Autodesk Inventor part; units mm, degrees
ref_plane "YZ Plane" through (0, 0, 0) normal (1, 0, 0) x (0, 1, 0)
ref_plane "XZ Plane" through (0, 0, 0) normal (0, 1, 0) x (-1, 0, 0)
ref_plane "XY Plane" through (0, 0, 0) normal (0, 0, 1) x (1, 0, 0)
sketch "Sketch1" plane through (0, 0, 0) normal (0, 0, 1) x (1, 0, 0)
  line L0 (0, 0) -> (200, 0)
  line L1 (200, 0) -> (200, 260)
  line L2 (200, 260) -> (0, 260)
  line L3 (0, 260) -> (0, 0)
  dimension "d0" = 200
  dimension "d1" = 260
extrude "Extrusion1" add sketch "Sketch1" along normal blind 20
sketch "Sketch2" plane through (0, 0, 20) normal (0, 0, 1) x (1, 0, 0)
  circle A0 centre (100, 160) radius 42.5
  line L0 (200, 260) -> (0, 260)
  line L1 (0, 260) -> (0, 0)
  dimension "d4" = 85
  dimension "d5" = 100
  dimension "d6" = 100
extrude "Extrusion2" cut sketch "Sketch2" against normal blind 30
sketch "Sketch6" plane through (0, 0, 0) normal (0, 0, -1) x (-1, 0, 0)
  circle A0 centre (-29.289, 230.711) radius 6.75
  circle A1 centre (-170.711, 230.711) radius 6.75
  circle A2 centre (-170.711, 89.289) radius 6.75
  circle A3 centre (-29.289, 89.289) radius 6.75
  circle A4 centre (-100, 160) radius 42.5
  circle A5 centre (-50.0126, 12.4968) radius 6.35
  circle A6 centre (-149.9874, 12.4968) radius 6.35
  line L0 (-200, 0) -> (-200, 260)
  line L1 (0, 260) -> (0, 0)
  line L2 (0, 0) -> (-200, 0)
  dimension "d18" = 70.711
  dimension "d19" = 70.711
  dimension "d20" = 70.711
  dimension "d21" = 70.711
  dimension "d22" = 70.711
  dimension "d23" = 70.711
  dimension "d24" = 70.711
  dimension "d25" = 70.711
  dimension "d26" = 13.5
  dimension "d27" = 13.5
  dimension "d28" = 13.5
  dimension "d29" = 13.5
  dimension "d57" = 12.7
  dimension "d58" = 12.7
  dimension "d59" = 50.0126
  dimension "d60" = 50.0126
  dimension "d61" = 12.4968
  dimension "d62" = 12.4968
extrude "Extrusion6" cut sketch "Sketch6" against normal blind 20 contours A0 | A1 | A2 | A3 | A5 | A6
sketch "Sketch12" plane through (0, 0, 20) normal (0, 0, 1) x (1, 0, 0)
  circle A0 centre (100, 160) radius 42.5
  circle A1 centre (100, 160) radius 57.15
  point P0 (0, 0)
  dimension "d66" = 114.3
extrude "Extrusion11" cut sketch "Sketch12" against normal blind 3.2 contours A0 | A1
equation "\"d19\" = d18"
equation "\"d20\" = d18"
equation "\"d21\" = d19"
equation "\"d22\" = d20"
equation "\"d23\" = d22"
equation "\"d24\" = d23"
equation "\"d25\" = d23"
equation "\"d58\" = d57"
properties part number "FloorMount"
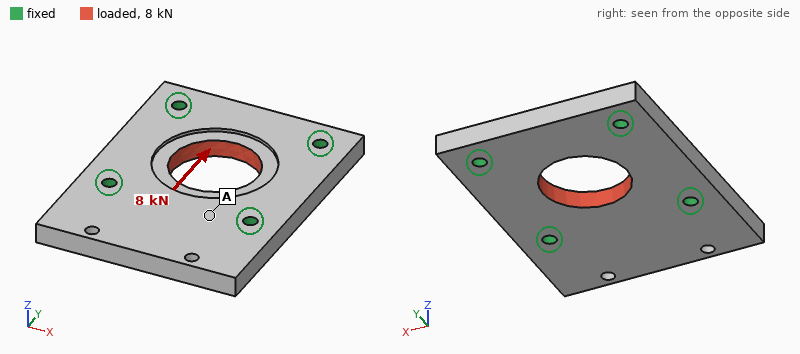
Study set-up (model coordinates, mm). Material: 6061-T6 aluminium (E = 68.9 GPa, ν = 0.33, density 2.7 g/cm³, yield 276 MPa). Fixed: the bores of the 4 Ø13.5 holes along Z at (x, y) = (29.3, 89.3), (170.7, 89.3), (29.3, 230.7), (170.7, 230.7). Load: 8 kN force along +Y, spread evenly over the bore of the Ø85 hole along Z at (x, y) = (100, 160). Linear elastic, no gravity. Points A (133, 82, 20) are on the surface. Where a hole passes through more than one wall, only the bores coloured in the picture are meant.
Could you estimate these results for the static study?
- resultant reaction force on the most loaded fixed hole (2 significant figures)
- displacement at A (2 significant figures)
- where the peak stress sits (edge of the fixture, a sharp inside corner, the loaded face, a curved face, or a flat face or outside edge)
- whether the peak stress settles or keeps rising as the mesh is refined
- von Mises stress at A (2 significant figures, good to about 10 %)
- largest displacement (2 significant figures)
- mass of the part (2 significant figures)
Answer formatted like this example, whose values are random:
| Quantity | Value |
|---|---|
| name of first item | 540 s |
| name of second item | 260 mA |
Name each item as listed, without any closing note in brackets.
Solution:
| Quantity | Value |
|---|---|
| resultant reaction force on the most loaded fixed hole | 2.1 kN |
| displacement at A | 1.2 µm |
| where the peak stress sits | edge of the fixture |
| whether the peak stress settles or keeps rising as the mesh is refined | keeps rising |
| von Mises stress at A | 0.81 MPa |
| largest displacement | 3.9 µm |
| mass of the part | 2.4 kg |
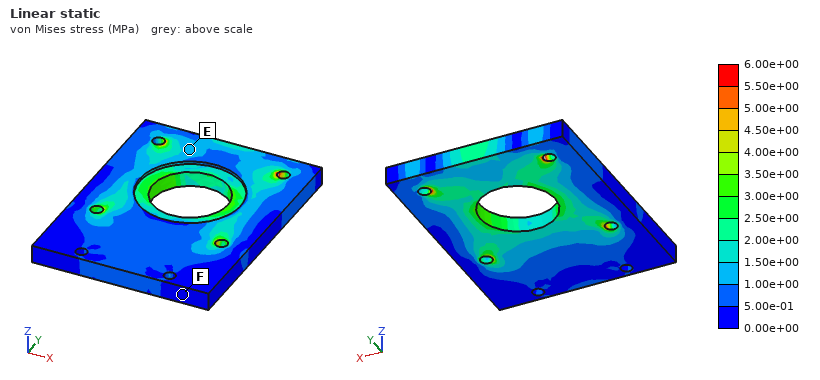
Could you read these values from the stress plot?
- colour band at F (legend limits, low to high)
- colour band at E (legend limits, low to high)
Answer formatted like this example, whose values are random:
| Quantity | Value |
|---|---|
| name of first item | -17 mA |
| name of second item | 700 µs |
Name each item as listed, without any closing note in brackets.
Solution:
| Quantity | Value |
|---|---|
| colour band at F | 0.00e+00 to 5.00e-01 MPa |
| colour band at E | 1.00e+00 to 1.50e+00 MPa |
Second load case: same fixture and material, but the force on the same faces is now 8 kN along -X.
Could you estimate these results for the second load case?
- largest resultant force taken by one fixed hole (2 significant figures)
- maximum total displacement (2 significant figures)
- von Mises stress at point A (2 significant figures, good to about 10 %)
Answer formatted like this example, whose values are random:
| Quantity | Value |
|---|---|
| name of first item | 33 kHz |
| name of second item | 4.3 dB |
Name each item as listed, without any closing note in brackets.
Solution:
| Quantity | Value |
|---|---|
| largest resultant force taken by one fixed hole | 2.1 kN |
| maximum total displacement | 3.7 µm |
| von Mises stress at point A | 1.1 MPa |
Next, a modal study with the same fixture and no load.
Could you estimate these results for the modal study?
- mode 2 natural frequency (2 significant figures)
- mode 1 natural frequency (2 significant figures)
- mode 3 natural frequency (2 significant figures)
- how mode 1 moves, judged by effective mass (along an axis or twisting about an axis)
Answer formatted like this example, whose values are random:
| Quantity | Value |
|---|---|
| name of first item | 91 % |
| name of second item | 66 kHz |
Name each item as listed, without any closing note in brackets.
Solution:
| Quantity | Value |
|---|---|
| mode 2 natural frequency | 2700 Hz |
| mode 1 natural frequency | 1700 Hz |
| mode 3 natural frequency | 3900 Hz |
| how mode 1 moves, judged by effective mass | along Z |
